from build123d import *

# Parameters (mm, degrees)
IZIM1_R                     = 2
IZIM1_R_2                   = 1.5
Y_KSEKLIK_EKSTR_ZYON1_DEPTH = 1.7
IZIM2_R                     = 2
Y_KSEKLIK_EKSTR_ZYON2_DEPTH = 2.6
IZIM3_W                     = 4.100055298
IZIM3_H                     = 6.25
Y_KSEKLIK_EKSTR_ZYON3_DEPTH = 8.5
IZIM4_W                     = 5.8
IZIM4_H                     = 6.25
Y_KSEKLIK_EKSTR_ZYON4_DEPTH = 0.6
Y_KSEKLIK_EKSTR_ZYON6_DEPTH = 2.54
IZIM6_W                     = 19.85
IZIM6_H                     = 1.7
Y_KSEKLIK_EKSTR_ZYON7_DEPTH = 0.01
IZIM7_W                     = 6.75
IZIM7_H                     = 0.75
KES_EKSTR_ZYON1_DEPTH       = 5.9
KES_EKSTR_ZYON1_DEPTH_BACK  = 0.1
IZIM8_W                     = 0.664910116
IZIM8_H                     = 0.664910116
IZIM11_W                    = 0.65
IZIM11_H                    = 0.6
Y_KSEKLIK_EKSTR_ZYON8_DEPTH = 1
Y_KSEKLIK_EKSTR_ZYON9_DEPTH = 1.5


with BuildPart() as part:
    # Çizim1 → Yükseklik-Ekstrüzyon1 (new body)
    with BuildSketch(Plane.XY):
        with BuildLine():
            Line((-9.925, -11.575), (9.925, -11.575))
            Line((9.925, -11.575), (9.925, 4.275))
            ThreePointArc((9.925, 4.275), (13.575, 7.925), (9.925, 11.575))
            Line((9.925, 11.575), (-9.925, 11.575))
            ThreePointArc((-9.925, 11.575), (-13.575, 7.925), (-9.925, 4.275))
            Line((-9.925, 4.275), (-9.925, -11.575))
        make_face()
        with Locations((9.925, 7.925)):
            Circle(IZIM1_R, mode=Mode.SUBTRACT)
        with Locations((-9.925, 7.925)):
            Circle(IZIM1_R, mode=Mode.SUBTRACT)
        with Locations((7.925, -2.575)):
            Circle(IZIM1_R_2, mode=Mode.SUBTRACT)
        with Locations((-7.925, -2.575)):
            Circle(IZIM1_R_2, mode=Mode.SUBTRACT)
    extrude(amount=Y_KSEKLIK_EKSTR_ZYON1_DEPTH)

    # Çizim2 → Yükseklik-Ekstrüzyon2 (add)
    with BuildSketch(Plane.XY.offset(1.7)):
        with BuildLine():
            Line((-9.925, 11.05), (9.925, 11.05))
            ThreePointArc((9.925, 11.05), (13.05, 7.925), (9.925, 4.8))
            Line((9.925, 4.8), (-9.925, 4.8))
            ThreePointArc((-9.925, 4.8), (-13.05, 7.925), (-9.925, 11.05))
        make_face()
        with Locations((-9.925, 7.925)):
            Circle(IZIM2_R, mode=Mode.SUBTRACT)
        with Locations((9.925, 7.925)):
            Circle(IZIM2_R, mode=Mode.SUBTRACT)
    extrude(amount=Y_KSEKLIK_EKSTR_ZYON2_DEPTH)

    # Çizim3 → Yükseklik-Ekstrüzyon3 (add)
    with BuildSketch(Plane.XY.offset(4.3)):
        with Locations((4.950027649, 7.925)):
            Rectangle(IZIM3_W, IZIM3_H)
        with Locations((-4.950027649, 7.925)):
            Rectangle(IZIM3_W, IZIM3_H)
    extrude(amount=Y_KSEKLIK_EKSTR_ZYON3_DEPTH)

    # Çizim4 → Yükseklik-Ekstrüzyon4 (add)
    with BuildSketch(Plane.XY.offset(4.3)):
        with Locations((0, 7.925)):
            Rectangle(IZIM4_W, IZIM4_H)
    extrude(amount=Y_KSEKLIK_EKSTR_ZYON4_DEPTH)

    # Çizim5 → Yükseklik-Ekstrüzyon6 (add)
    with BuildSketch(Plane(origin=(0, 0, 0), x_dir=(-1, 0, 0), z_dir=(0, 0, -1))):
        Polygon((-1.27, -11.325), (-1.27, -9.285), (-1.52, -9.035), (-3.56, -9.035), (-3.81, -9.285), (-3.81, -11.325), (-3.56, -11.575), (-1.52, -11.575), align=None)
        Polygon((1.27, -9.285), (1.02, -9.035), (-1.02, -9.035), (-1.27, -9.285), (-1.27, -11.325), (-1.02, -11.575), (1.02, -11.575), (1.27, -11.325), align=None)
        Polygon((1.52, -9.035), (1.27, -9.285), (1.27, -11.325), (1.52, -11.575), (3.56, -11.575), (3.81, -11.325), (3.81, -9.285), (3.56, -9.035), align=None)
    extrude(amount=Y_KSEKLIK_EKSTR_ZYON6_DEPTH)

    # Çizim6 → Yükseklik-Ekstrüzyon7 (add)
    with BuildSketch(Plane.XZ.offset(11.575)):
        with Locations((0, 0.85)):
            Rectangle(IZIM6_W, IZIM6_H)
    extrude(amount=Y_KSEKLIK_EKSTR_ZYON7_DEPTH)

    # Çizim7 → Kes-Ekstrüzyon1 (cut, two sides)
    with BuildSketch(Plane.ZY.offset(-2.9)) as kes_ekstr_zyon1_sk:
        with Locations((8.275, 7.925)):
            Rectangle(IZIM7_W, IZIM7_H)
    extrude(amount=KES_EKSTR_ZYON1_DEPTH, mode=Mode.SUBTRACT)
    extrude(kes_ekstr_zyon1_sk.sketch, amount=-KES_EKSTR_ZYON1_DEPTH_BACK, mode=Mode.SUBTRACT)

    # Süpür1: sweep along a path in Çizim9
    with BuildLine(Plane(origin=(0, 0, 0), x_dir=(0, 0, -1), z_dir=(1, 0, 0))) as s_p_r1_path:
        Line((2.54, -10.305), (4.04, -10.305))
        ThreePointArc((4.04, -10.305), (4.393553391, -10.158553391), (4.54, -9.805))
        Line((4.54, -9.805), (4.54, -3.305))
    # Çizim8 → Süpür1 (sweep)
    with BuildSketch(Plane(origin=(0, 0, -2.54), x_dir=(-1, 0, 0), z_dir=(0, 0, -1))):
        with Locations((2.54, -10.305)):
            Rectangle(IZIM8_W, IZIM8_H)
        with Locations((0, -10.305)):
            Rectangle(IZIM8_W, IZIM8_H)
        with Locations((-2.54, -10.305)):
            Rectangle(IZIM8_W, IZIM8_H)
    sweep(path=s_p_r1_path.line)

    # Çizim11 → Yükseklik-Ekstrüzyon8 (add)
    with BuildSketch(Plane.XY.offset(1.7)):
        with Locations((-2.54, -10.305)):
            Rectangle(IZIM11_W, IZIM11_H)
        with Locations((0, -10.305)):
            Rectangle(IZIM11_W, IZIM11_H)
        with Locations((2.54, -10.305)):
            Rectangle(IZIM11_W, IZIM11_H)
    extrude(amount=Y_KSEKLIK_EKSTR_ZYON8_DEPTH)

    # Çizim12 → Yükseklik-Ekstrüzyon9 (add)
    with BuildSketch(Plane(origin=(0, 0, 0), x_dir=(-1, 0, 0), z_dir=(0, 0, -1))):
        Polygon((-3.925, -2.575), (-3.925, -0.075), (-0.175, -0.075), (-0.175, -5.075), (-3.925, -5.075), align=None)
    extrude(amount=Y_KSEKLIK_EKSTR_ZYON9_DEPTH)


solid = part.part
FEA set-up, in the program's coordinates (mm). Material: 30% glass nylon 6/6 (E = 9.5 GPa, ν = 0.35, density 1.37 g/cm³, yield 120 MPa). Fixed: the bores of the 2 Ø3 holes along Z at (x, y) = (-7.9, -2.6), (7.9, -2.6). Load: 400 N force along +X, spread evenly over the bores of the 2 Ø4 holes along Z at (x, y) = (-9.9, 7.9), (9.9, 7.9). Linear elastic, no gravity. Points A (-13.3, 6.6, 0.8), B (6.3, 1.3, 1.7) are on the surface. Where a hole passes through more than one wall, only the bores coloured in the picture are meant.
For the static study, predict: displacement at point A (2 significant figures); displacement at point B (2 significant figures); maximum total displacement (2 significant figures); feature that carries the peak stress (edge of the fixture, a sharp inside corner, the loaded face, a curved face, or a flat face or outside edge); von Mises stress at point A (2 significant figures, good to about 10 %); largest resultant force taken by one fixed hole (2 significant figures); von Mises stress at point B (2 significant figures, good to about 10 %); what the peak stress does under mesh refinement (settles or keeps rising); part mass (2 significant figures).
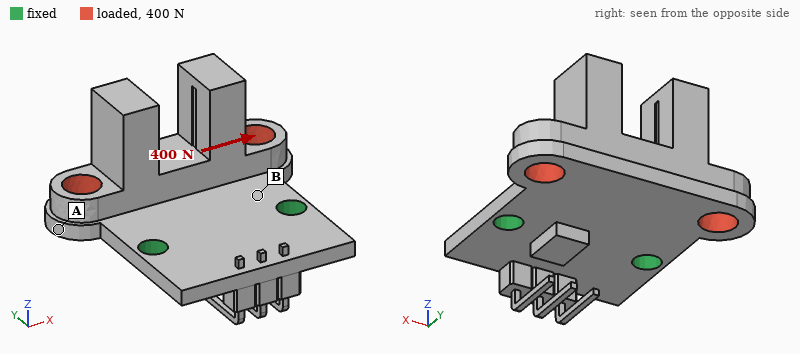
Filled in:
0.099 mm
0.020 mm
0.12 mm
edge of the fixture
9.9 MPa
320 N
38 MPa
keeps rising
2.3 g
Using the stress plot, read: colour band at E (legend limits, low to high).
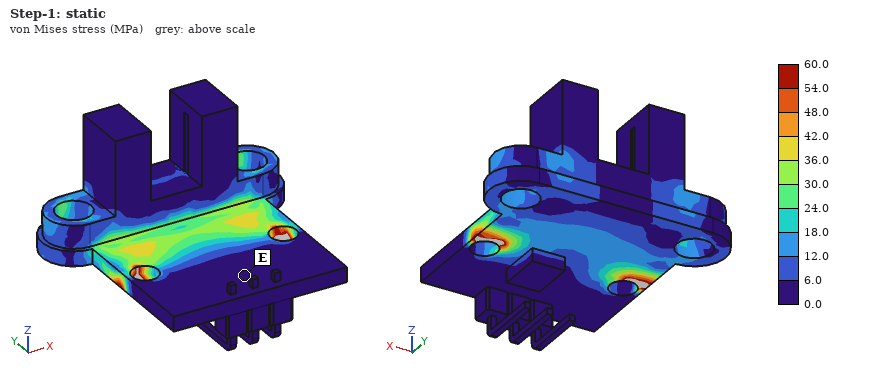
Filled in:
0.0 to 6.0 MPa
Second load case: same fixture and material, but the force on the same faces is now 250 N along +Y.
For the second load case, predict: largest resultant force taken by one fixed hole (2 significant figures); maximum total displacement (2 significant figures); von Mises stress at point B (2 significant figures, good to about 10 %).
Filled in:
130 N
0.44 mm
41 MPa
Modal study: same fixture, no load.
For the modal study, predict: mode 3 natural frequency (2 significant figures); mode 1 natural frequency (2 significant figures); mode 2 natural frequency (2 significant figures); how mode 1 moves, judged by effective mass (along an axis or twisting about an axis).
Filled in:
3500 Hz
1600 Hz
3500 Hz
along Z
